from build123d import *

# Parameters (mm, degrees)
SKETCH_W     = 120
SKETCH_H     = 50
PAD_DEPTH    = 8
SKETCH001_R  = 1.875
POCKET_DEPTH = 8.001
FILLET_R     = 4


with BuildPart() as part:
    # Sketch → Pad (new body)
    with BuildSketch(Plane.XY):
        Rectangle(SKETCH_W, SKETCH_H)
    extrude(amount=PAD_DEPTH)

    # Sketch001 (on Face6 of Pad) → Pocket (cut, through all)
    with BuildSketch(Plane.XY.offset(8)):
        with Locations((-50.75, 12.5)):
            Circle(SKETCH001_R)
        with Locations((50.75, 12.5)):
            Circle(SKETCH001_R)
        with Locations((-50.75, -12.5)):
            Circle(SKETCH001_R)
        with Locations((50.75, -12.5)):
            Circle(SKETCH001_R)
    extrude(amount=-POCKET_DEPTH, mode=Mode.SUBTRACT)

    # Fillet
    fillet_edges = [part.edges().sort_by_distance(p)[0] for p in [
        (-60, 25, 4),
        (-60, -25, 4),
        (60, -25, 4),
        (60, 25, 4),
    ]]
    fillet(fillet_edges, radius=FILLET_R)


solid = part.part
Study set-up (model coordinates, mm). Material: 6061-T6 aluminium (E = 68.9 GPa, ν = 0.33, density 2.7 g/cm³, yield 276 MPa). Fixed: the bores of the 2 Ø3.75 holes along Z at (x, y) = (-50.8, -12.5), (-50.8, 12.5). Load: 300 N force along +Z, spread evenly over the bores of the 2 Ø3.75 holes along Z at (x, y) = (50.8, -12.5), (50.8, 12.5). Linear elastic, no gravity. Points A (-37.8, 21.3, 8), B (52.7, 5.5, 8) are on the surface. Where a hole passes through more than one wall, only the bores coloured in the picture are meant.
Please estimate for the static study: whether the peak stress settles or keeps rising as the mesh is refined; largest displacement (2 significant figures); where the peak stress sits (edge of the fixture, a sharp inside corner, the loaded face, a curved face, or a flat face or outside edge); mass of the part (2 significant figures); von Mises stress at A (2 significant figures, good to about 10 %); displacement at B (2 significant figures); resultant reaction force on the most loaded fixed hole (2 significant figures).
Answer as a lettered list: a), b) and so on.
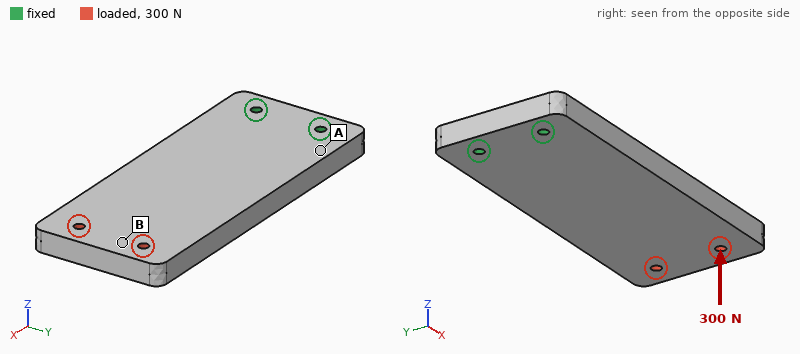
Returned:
a) keeps rising
b) 0.85 mm
c) edge of the fixture
d) 130 g
e) 48 MPa
f) 0.77 mm
g) 150 N
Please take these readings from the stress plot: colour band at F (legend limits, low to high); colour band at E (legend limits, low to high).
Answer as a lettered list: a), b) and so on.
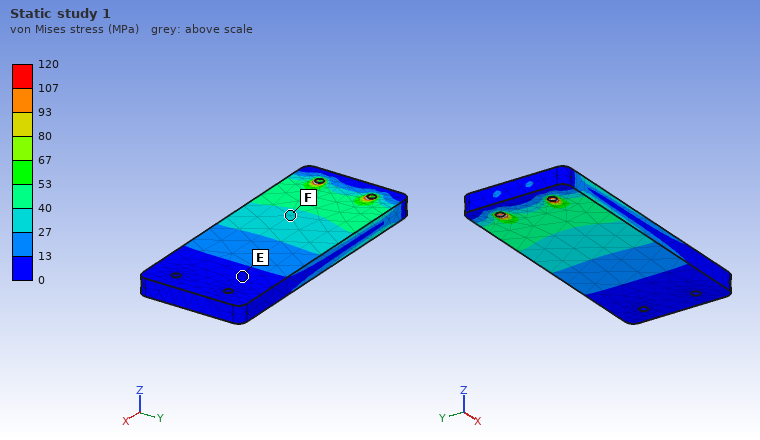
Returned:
a) 27 to 40 MPa
b) 0 to 13 MPa
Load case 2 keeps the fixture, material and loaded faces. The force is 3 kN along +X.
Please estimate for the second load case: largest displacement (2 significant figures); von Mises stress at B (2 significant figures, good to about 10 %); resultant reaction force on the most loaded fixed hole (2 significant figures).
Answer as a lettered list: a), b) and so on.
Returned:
a) 13 µm
b) 5.1 MPa
c) 1.5 kN
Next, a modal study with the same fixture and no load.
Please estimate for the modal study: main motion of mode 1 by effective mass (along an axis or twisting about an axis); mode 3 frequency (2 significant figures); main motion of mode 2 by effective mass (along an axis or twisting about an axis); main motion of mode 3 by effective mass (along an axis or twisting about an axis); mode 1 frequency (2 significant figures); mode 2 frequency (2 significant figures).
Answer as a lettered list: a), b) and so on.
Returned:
a) along Z
b) 2400 Hz
c) twisting about X
d) along Y
e) 520 Hz
f) 2300 Hz
